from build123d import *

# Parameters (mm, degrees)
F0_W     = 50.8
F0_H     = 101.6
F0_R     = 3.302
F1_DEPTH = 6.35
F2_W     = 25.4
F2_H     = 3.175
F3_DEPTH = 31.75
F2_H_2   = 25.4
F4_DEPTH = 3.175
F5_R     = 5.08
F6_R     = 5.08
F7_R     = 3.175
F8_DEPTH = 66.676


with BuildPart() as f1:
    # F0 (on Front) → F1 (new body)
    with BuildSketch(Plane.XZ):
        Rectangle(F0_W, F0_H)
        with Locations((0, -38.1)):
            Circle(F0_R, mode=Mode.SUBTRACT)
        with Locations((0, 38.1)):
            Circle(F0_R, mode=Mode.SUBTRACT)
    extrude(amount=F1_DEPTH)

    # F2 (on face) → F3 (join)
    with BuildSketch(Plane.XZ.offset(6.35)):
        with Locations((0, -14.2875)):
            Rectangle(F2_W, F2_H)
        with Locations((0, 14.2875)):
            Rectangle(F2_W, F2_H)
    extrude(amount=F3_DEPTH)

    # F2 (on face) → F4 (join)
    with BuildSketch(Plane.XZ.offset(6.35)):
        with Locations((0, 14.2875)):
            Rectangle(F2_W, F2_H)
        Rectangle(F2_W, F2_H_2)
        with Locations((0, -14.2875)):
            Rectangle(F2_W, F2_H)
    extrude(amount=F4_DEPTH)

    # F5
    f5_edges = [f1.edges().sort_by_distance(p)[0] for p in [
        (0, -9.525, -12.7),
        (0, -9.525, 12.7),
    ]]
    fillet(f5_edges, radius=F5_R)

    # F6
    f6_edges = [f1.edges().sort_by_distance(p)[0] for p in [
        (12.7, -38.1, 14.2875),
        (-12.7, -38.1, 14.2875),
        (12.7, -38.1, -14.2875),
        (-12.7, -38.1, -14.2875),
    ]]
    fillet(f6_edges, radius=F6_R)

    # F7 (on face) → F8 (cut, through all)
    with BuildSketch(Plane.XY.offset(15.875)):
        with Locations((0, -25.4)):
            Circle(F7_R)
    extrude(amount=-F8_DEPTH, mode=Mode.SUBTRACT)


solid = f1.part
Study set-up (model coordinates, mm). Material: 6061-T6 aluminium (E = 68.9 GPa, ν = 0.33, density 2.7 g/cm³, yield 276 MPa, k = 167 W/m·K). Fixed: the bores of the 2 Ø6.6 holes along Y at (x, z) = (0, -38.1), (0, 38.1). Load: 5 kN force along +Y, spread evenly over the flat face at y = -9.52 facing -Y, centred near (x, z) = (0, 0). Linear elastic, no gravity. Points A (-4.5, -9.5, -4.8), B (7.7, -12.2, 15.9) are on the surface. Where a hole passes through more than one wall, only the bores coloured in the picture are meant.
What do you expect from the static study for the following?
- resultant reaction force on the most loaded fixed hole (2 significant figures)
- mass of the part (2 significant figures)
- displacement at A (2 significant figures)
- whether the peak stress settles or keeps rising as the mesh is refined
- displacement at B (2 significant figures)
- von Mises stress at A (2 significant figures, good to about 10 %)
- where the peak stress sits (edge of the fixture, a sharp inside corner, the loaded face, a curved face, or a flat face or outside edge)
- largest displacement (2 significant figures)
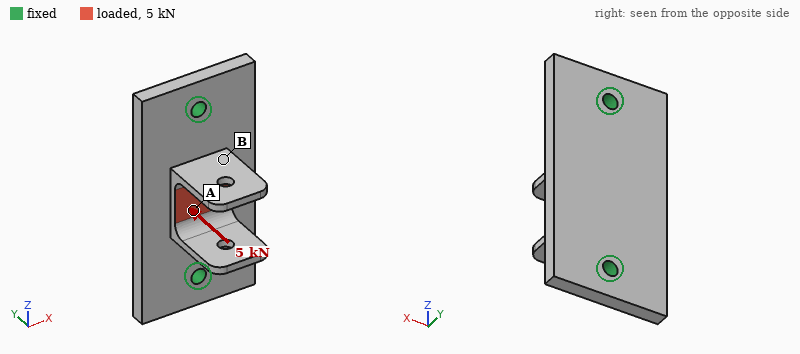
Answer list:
2.8 kN
110 g
0.12 mm
keeps rising
0.099 mm
81 MPa
edge of the fixture
0.14 mm
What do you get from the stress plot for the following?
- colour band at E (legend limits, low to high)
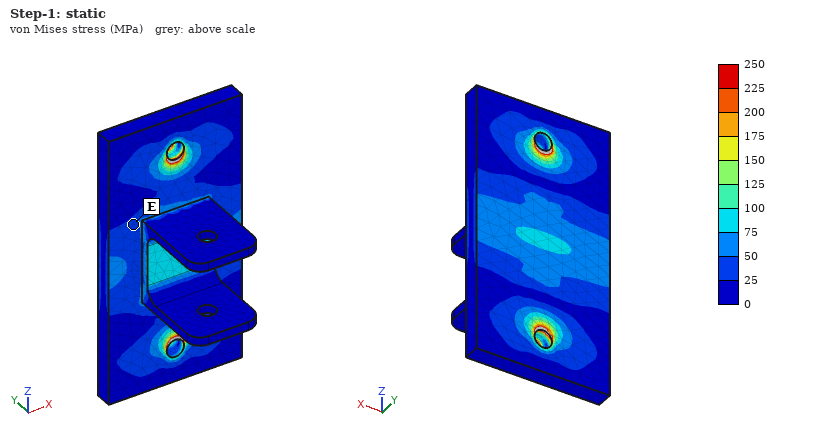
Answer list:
25 to 50 MPa
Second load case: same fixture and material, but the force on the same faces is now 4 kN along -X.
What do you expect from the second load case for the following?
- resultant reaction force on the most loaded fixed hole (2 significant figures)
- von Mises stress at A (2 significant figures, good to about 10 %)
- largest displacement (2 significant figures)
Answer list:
2.0 kN
25 MPa
0.11 mm
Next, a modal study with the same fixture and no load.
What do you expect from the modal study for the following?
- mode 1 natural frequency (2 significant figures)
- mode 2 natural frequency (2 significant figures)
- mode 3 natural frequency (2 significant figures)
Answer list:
3500 Hz
3500 Hz
3600 Hz
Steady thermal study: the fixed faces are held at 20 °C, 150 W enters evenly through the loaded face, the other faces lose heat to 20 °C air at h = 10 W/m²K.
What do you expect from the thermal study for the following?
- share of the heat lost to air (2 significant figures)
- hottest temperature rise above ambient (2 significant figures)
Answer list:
3.2 %
66 K
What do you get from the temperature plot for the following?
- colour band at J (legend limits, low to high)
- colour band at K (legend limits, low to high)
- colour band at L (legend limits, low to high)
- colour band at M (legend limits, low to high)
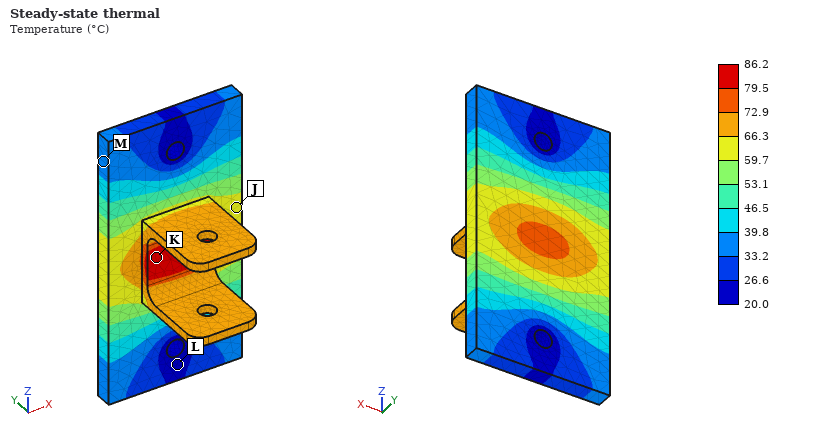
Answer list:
59.7 to 66.3 °C
79.5 to 86.2 °C
20.0 to 26.6 °C
33.2 to 39.8 °C
